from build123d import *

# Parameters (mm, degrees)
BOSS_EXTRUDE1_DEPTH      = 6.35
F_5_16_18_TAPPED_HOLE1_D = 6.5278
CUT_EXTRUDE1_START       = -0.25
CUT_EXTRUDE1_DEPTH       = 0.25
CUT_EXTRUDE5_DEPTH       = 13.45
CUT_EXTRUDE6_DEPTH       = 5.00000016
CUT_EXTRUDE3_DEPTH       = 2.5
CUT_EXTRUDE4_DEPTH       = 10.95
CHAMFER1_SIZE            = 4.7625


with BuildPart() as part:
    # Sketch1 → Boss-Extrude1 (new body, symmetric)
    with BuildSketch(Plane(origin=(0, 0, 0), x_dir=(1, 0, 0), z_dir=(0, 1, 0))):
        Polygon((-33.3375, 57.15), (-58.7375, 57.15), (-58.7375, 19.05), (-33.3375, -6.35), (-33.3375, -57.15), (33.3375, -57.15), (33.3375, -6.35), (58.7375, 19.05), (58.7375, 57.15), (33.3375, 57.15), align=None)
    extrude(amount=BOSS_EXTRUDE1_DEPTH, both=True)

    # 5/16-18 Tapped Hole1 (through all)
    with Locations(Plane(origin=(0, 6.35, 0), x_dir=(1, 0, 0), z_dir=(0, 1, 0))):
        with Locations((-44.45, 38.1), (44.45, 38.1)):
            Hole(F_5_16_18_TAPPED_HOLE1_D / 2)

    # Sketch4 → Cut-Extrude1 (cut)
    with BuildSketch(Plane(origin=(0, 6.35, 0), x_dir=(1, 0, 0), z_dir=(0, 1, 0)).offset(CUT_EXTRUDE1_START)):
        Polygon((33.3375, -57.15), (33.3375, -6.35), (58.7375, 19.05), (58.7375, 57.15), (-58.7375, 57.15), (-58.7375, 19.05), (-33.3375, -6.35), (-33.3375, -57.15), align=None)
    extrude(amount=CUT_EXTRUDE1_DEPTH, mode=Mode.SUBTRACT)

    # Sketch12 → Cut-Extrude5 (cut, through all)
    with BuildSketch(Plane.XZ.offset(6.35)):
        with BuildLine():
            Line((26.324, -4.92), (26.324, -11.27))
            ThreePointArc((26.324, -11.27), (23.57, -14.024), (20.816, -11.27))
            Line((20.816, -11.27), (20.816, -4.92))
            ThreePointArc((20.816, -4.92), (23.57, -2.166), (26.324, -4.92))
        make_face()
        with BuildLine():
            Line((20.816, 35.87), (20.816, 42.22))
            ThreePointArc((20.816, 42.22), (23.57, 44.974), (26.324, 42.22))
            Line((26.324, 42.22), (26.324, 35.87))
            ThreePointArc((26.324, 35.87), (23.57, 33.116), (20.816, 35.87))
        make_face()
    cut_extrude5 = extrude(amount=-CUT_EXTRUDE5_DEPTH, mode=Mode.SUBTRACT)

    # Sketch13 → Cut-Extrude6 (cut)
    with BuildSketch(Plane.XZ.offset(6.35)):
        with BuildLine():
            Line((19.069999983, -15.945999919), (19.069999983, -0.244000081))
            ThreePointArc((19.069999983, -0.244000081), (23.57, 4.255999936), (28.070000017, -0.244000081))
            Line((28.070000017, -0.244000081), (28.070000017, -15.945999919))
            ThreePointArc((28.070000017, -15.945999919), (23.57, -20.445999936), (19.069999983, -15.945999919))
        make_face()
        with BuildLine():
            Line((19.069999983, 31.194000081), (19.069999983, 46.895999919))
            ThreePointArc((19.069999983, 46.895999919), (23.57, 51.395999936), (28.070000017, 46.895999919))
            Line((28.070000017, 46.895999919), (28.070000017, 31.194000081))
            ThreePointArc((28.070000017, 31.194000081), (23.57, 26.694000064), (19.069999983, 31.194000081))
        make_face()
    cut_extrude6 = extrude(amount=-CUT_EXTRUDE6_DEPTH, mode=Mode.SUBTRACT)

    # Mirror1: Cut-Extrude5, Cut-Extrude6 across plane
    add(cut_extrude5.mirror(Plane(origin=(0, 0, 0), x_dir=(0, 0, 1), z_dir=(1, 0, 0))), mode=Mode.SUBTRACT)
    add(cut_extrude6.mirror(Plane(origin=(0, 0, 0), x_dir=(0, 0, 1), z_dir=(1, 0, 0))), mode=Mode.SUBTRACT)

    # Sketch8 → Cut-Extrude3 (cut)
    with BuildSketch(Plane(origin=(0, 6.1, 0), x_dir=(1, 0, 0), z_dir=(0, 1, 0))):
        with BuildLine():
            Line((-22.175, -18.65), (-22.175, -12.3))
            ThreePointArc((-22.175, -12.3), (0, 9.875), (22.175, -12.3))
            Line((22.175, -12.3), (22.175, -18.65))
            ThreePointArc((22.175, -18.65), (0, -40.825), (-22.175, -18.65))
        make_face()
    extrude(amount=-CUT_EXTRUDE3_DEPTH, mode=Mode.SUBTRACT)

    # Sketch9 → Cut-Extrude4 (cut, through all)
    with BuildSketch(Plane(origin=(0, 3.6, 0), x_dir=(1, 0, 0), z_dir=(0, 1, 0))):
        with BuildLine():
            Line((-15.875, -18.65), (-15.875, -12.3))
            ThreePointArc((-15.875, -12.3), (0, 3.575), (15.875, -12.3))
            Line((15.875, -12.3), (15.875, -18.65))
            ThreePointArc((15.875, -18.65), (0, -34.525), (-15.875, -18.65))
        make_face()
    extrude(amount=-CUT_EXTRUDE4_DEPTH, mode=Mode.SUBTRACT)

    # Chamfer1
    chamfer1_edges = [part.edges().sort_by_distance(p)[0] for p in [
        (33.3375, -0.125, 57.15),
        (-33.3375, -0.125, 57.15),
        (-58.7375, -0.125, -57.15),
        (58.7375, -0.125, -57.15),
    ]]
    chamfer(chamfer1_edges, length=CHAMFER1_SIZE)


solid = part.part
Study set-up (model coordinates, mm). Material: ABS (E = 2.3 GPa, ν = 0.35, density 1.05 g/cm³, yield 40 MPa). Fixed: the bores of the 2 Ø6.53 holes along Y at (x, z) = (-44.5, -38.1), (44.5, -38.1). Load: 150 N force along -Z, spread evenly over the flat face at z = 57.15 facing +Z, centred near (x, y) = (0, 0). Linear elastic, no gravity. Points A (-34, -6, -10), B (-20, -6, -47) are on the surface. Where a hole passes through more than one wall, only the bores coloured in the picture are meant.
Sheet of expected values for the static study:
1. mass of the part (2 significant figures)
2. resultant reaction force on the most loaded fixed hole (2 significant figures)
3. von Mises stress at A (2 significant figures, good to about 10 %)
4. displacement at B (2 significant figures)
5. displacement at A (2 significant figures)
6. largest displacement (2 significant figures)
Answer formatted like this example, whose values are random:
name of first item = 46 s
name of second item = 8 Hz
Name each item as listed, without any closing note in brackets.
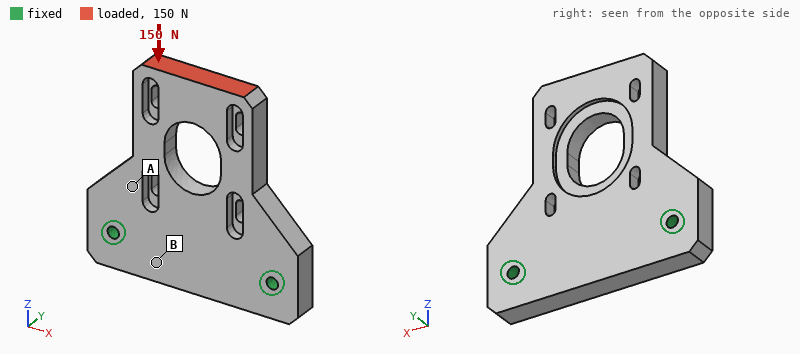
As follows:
mass of the part = 110 g
resultant reaction force on the most loaded fixed hole = 78 N
von Mises stress at A = 0.29 MPa
displacement at B = 3.0 µm
displacement at A = 3.6 µm
largest displacement = 17 µm
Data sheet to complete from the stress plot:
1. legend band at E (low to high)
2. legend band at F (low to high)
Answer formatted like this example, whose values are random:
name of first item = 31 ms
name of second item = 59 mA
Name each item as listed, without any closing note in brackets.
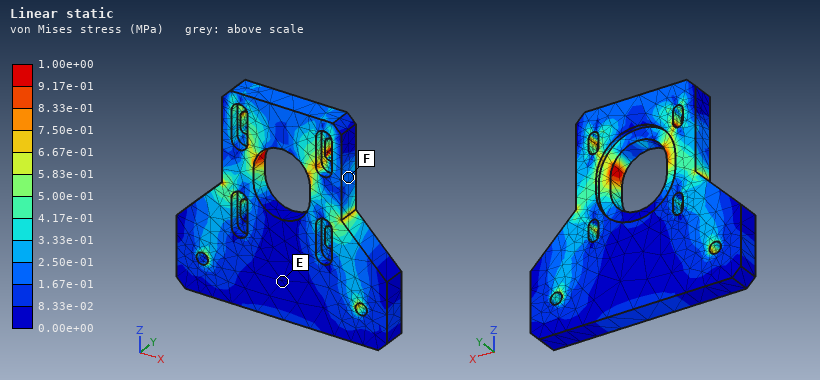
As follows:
legend band at E = 0.00e+00 to 8.33e-02 MPa
legend band at F = 1.67e-01 to 2.50e-01 MPa
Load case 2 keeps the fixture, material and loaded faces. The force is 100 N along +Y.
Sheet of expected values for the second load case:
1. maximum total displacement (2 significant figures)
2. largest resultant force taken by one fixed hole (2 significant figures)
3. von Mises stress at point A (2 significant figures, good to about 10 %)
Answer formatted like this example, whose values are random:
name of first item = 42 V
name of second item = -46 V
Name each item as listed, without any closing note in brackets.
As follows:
maximum total displacement = 1.7 mm
largest resultant force taken by one fixed hole = 50 N
von Mises stress at point A = 4.8 MPa
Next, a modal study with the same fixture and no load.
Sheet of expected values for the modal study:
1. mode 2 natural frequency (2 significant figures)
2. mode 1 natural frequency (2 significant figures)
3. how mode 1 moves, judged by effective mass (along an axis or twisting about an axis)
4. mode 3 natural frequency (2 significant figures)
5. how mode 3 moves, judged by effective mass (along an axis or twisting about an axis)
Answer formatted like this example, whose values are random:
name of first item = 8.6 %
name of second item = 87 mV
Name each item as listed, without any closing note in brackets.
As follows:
mode 2 natural frequency = 900 Hz
mode 1 natural frequency = 320 Hz
how mode 1 moves, judged by effective mass = along Y
mode 3 natural frequency = 1400 Hz
how mode 3 moves, judged by effective mass = along Y
